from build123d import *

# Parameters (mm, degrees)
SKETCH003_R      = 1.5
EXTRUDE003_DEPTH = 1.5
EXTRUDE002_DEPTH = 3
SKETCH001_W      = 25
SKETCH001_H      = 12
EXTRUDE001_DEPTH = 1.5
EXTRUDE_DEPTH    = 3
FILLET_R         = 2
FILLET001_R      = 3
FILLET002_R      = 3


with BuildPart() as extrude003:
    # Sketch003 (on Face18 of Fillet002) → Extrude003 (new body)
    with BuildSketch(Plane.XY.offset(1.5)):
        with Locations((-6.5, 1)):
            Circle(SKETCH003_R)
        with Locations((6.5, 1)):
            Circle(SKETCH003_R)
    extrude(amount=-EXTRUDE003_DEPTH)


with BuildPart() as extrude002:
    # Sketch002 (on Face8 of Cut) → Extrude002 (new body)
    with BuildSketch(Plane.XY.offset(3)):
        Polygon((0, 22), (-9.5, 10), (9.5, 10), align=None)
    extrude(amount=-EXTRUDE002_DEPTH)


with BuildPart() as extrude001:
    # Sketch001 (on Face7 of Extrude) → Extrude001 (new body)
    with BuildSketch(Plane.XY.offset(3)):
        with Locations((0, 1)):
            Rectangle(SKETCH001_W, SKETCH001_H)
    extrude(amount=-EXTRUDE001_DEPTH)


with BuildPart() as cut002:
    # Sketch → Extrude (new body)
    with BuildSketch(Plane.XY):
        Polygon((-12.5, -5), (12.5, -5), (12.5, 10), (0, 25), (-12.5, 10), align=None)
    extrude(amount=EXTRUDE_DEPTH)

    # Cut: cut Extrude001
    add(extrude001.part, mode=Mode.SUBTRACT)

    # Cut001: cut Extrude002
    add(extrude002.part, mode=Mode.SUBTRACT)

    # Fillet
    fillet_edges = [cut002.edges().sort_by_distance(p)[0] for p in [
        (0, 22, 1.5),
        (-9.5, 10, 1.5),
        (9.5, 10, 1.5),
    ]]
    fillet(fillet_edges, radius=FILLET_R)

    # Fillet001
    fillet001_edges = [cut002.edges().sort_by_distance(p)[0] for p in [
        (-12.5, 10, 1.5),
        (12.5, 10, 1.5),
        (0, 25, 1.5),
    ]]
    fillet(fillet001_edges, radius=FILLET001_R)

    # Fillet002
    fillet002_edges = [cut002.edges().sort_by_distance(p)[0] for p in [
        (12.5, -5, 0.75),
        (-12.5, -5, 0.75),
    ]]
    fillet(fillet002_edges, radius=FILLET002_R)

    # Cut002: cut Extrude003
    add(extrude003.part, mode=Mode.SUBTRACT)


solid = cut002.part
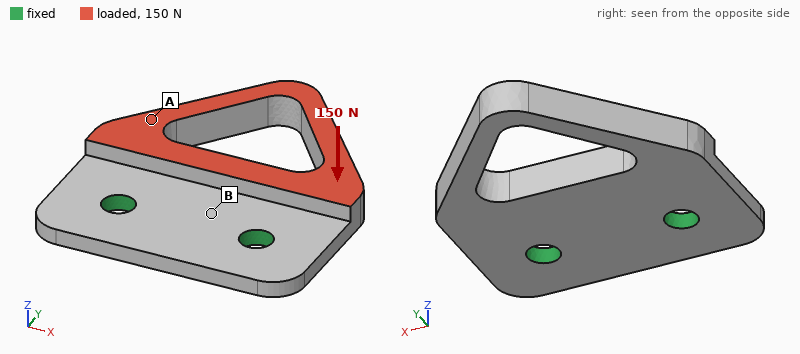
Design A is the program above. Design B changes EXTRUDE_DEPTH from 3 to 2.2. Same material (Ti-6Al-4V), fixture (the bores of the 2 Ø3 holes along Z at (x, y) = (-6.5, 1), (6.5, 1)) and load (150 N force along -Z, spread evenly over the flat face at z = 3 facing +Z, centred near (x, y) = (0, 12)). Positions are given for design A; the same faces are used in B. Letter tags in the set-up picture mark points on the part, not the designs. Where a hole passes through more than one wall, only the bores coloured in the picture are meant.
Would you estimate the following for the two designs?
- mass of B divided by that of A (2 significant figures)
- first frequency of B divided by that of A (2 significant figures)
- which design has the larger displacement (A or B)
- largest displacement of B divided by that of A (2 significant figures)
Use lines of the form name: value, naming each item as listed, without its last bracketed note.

mass of B divided by that of A: 0.86
first frequency of B divided by that of A: 1.1
which design has the larger displacement: B
largest displacement of B divided by that of A: 1.2
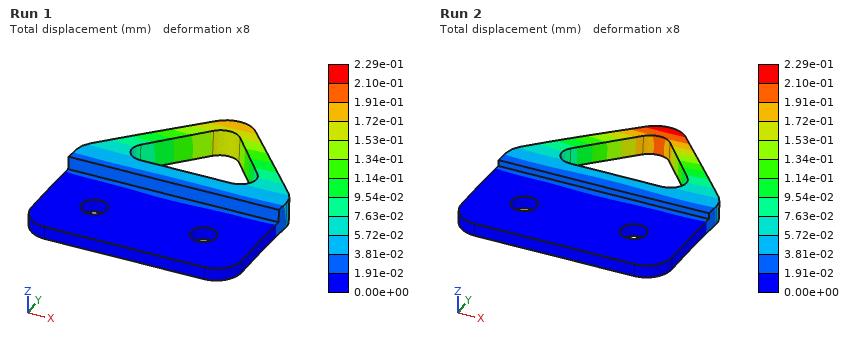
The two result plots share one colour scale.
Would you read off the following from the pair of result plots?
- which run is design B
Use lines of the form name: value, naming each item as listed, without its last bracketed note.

which run is design B: Run 2
